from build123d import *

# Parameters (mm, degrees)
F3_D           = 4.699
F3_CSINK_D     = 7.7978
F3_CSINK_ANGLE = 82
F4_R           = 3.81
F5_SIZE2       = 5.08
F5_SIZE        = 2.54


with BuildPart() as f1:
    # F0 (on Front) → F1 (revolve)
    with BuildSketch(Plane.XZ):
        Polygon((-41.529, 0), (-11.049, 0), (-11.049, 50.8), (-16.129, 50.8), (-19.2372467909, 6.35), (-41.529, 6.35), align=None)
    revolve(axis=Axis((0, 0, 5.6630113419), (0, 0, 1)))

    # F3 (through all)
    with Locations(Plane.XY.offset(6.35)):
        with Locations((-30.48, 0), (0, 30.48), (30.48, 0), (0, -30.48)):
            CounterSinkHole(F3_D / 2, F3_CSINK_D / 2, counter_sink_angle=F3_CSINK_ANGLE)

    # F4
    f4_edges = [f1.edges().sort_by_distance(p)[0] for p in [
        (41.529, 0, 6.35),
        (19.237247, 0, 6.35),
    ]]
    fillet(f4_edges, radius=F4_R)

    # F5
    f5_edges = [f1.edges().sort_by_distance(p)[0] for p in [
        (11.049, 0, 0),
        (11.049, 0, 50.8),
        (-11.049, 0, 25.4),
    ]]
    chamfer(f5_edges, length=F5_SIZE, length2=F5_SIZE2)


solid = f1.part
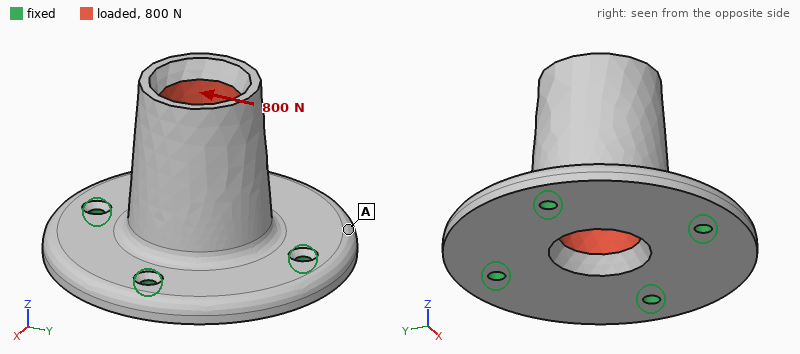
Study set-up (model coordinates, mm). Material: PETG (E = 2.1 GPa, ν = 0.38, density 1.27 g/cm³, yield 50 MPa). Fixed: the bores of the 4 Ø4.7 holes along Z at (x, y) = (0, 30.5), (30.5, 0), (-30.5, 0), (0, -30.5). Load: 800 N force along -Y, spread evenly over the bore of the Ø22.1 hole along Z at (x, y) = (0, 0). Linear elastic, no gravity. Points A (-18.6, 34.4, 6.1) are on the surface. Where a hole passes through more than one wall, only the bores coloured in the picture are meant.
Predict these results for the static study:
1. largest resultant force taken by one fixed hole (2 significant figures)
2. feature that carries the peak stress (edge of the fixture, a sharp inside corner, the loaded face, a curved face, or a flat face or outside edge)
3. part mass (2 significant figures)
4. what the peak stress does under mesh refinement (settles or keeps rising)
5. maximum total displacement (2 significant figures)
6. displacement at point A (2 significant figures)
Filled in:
440 N
edge of the fixture
72 g
keeps rising
0.31 mm
0.047 mm
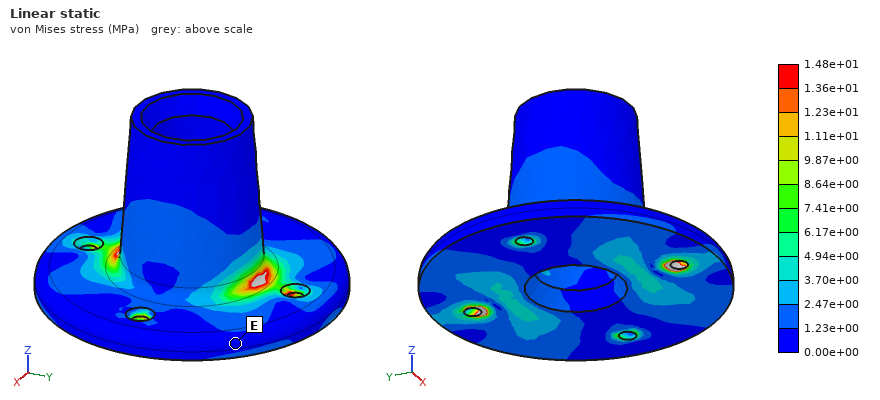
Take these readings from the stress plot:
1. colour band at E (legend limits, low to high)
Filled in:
0.00e+00 to 1.23e+00 MPa
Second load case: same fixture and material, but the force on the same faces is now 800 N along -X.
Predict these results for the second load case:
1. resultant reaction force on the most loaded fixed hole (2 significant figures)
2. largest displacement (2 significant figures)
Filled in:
440 N
0.31 mm
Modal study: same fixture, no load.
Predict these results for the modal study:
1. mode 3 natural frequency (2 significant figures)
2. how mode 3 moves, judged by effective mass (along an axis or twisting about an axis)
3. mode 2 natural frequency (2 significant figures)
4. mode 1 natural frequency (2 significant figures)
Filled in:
2200 Hz
along Z
1600 Hz
1600 Hz
